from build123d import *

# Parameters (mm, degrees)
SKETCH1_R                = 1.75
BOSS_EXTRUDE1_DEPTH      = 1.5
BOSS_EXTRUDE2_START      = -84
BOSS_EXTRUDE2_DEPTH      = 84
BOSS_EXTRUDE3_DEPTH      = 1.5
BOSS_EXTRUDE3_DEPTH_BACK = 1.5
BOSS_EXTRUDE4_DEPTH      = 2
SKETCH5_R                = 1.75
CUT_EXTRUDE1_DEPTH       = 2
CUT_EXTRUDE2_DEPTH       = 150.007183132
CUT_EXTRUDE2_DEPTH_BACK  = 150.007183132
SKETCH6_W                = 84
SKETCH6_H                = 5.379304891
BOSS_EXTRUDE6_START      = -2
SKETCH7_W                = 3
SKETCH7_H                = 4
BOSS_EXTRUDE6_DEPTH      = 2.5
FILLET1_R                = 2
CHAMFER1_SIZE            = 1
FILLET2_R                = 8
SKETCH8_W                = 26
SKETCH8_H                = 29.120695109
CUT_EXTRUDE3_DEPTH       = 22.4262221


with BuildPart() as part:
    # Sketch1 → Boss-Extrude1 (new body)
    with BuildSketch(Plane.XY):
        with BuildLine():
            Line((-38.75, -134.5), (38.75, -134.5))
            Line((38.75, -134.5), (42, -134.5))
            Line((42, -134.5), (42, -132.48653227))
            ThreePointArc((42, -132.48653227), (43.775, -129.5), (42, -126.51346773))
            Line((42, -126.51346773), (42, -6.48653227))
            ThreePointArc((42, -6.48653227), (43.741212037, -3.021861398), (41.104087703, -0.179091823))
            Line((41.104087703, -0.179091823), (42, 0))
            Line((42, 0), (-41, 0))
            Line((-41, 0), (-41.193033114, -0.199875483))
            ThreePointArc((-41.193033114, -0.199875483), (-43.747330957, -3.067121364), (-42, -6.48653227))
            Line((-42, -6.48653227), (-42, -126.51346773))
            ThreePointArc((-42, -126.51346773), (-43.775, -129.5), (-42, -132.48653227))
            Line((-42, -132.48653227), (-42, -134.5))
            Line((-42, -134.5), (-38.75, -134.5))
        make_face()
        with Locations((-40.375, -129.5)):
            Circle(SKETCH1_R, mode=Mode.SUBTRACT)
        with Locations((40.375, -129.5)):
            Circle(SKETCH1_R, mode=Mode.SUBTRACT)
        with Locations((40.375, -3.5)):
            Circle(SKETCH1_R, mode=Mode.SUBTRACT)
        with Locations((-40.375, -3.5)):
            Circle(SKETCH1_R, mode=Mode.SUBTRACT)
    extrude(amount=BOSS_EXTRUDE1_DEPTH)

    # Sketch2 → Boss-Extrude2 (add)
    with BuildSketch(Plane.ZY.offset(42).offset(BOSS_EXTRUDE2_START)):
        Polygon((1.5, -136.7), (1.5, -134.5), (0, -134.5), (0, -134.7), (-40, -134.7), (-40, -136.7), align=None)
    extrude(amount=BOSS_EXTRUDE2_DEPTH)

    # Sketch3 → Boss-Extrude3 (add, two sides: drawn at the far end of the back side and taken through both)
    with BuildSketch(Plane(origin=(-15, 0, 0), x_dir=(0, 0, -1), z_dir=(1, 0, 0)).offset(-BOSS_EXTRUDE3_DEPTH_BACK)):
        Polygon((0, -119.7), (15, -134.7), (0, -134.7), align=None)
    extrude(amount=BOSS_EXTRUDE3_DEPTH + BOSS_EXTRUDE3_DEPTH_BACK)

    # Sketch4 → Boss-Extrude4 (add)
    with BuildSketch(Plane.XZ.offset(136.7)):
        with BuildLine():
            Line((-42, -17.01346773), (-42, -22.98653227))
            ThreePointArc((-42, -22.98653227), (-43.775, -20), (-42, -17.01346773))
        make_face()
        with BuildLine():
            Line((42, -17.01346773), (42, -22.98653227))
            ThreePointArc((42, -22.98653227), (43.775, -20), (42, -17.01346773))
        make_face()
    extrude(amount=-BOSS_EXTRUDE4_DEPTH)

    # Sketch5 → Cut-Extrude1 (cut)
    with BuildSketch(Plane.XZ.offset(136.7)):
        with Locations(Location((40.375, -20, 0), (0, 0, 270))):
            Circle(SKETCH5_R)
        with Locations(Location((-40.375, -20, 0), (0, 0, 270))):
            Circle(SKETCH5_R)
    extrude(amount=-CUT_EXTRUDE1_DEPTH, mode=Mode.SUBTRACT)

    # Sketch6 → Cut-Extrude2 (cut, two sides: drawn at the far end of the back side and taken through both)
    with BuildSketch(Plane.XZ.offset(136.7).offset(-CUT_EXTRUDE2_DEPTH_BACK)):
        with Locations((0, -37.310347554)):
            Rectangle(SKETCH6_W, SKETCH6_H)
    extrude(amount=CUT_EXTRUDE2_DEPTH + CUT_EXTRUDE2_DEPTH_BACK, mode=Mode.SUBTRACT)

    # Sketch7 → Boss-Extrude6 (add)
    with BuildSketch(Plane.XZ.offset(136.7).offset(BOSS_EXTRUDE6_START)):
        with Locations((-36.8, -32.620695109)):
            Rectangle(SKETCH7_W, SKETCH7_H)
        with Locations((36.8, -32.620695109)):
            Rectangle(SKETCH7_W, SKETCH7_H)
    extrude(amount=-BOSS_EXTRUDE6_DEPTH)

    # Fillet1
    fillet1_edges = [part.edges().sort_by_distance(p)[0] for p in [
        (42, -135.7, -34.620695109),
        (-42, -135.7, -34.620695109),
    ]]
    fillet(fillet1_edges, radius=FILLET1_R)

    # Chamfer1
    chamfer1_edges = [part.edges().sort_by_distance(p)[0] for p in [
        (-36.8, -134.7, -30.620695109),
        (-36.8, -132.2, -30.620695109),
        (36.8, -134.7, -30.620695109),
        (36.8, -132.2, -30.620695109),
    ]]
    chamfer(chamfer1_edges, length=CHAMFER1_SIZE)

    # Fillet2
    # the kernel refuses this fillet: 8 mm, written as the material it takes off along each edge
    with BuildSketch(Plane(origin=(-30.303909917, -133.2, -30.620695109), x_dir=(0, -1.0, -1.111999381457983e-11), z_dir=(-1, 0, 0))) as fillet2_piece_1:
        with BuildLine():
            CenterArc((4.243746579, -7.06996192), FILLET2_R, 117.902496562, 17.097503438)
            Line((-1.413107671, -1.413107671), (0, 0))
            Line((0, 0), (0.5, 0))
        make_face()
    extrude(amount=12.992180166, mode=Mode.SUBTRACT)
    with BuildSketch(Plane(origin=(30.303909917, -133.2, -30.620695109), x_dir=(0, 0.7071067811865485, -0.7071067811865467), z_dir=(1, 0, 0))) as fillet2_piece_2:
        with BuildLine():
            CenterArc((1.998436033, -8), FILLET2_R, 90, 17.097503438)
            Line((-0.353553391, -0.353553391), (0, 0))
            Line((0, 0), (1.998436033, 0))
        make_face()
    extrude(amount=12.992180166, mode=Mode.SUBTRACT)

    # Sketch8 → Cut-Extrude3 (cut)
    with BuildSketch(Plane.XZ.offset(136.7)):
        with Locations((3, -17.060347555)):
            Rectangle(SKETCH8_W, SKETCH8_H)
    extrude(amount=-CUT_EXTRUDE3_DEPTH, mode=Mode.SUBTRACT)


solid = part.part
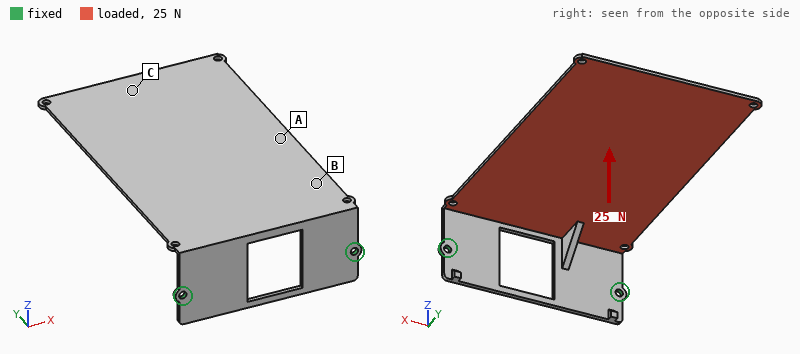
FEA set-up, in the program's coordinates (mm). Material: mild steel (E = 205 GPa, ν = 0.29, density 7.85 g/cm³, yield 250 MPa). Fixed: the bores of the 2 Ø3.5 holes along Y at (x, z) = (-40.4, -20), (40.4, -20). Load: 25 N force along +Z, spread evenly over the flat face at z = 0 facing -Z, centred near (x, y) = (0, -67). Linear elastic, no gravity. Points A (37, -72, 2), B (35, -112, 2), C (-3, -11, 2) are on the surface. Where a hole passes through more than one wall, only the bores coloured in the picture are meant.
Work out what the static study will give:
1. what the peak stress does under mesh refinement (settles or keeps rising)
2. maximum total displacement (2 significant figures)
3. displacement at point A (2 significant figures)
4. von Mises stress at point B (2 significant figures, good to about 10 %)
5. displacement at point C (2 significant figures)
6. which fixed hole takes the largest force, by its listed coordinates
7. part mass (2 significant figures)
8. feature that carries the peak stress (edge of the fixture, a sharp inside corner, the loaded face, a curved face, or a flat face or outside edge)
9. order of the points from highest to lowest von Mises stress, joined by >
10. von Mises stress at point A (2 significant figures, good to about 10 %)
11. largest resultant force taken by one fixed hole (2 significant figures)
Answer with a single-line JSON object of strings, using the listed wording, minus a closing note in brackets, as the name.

{"what the peak stress does under mesh refinement": "keeps rising", "maximum total displacement": "1.9 mm", "displacement at point A": "0.65 mm", "von Mises stress at point B": "29 MPa", "displacement at point C": "1.7 mm", "which fixed hole takes the largest force, by its listed coordinates": "(-40.4, -20)", "part mass": "170 g", "feature that carries the peak stress": "edge of the fixture", "order of the points from highest to lowest von Mises stress, joined by >": "B > A > C", "von Mises stress at point A": "15 MPa", "largest resultant force taken by one fixed hole": "17 N"}
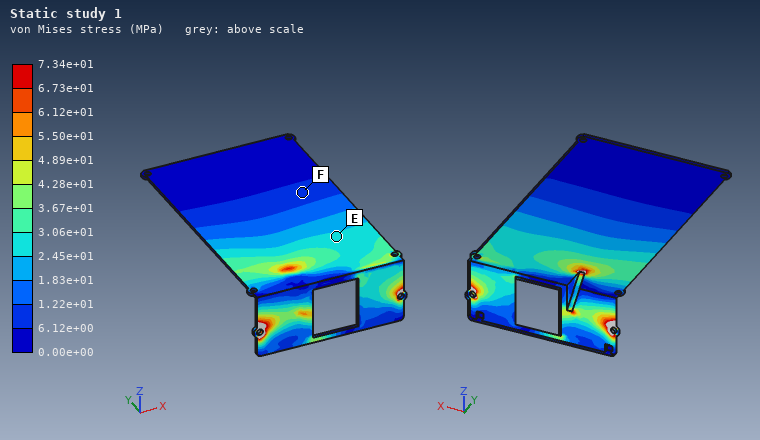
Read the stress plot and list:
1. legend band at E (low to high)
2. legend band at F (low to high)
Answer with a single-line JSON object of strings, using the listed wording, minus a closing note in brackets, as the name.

{"legend band at E": "2.45e+01 to 3.06e+01 MPa", "legend band at F": "6.12e+00 to 1.22e+01 MPa"}
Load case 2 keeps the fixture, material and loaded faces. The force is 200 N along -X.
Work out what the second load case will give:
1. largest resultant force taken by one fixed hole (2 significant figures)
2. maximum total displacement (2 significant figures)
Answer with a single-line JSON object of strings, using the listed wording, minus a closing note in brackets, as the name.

{"largest resultant force taken by one fixed hole": "220 N", "maximum total displacement": "0.73 mm"}
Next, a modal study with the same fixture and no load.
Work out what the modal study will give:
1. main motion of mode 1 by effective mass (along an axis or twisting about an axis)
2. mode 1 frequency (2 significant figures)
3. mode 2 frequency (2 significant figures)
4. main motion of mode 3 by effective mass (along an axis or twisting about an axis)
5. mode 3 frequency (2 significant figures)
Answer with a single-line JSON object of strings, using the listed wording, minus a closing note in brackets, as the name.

{"main motion of mode 1 by effective mass": "along Z", "mode 1 frequency": "63 Hz", "mode 2 frequency": "230 Hz", "main motion of mode 3 by effective mass": "along X", "mode 3 frequency": "320 Hz"}
